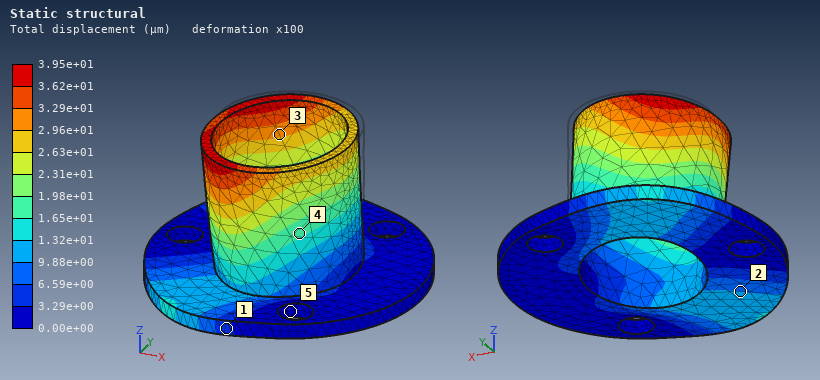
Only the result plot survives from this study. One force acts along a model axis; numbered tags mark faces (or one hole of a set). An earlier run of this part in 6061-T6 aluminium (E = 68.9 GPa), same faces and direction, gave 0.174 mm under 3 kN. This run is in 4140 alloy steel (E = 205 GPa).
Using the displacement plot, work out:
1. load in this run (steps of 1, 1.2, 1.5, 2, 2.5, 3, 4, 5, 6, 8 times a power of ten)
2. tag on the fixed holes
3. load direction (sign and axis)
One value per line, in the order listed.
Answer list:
2 kN
5
-Y
